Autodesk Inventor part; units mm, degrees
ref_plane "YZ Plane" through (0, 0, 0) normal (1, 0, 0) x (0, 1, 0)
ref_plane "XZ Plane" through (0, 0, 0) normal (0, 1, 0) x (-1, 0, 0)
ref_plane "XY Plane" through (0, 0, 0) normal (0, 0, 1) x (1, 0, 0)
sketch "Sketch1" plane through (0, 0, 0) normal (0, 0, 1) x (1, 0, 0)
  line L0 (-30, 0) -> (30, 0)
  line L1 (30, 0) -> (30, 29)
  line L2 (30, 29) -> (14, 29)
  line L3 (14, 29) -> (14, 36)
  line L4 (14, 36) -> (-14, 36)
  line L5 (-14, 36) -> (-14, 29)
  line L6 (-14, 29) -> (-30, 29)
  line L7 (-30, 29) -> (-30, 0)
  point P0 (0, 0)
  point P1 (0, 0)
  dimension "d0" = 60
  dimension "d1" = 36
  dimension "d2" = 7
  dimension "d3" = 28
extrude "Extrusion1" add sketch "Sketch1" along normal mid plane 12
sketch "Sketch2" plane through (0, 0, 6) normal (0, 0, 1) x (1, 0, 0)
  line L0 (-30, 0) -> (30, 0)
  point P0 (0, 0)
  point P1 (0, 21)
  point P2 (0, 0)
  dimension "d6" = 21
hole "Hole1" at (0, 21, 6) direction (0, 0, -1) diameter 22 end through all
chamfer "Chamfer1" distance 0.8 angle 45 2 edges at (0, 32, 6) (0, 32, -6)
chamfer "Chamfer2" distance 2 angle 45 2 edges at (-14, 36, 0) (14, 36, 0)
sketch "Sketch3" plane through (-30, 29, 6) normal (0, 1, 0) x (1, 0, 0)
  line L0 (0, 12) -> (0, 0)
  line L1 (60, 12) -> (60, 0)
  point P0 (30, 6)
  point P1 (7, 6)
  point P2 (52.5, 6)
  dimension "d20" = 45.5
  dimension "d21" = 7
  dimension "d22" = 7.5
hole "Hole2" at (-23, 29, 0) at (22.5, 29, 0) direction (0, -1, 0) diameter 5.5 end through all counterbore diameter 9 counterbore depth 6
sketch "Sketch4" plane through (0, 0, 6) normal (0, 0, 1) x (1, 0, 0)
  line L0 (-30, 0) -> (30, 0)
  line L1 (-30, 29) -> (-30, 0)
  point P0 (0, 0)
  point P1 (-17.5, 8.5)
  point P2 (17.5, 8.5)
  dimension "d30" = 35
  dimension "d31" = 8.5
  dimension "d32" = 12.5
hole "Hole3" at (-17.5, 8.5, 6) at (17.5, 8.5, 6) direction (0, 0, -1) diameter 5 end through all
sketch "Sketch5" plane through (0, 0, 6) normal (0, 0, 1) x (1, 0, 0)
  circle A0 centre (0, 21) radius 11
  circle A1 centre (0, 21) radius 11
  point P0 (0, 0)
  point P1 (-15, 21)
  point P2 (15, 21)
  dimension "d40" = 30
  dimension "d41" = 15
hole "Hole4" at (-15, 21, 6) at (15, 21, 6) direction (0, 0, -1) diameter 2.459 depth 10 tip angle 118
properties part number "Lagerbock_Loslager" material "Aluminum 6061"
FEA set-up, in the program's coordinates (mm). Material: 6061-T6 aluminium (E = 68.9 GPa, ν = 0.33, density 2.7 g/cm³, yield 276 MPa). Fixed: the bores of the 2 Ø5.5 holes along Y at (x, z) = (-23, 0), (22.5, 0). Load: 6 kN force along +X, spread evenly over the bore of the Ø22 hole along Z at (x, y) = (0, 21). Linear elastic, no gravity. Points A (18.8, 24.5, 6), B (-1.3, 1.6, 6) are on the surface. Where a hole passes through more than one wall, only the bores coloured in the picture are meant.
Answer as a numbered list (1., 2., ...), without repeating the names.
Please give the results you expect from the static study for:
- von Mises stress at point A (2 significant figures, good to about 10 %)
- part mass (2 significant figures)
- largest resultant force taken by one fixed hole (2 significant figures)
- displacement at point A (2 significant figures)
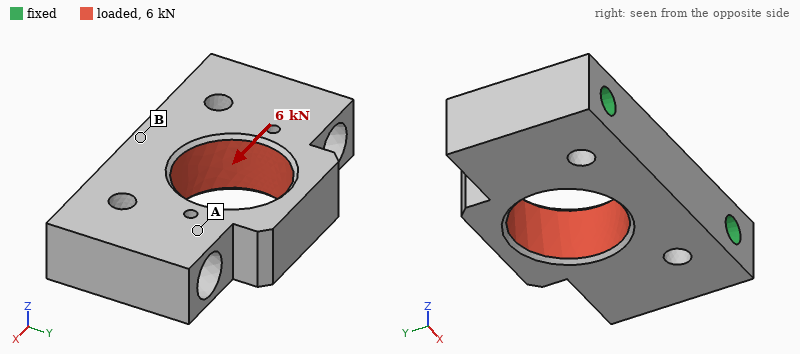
1. 19 MPa
2. 44 g
3. 3.0 kN
4. 3.5 µm
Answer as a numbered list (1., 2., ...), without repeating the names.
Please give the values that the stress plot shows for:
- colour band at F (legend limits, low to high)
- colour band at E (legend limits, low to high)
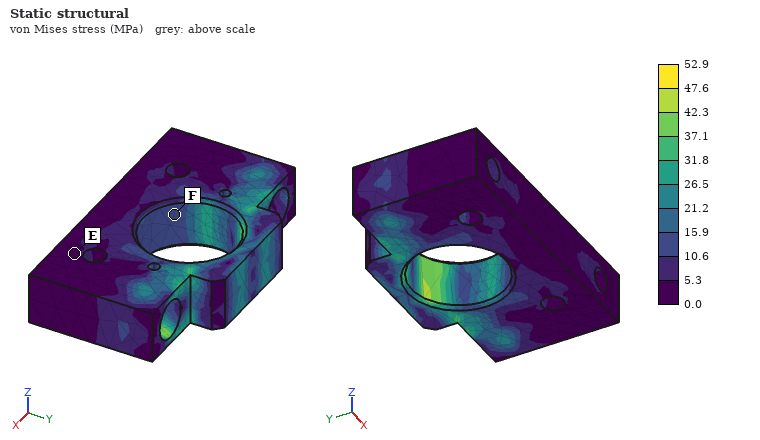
1. 10.6 to 15.9 MPa
2. 0.0 to 5.3 MPa
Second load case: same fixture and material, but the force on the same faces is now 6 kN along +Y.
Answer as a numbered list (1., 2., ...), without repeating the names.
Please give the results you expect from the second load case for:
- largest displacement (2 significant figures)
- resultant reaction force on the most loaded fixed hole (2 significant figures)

1. 14 µm
2. 3.1 kN
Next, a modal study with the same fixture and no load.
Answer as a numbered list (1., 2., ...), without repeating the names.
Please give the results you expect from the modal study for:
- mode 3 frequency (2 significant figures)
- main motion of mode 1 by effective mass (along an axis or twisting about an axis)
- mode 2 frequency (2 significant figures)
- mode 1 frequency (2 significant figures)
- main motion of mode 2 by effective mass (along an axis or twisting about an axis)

1. 27 kHz
2. along Z
3. 22 kHz
4. 15 kHz
5. along Z
